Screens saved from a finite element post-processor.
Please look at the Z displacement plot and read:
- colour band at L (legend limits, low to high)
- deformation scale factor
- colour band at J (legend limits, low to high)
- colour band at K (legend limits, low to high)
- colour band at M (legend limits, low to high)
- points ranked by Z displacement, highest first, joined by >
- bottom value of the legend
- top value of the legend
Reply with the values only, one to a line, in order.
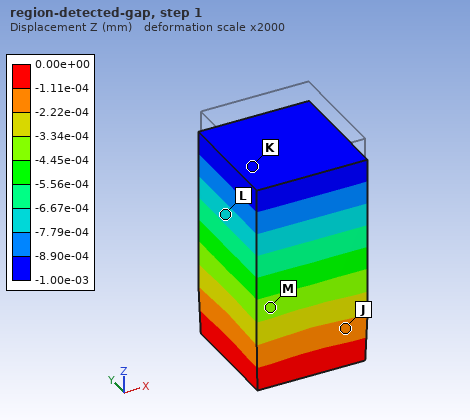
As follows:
-7.79e-04 to -6.67e-04 mm
2000
-2.22e-04 to -1.11e-04 mm
-1.00e-03 to -8.90e-04 mm
-4.45e-04 to -3.34e-04 mm
J > M > L > K
-1.00e-03 mm
0.00e+00 mm
